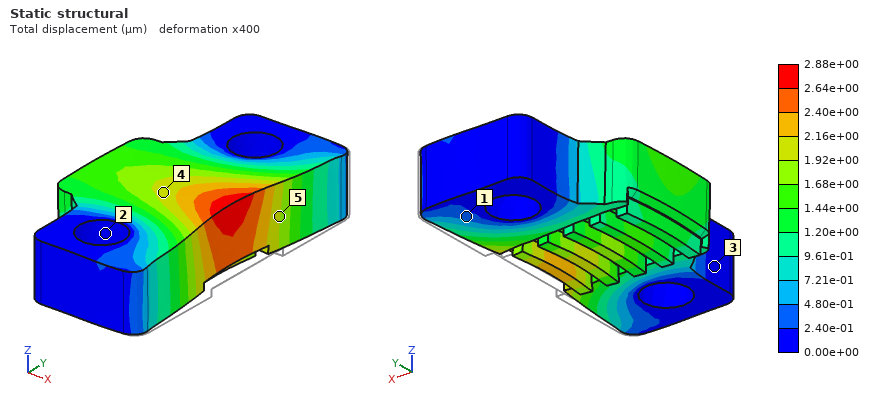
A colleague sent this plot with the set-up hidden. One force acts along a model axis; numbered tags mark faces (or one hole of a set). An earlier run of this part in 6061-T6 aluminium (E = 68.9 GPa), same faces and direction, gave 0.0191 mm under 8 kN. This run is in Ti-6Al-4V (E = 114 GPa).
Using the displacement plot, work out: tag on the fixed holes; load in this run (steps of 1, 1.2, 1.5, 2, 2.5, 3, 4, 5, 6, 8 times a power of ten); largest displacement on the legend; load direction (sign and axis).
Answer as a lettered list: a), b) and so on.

a) 2
b) 2 kN
c) 2.88e+00 µm
d) -X
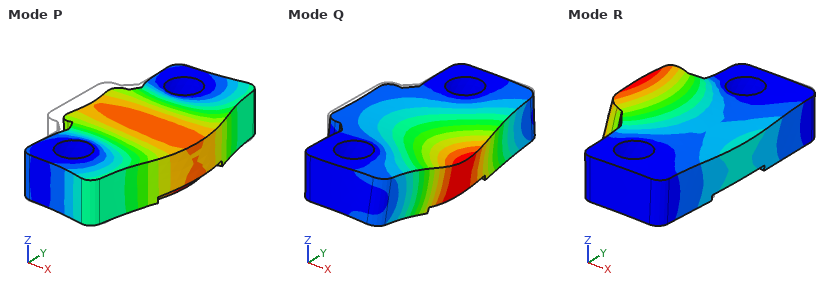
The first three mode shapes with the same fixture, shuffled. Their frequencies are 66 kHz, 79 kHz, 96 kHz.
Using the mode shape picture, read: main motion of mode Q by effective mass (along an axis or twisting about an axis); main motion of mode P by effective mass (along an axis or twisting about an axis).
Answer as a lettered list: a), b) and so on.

a) along Z
b) along X
